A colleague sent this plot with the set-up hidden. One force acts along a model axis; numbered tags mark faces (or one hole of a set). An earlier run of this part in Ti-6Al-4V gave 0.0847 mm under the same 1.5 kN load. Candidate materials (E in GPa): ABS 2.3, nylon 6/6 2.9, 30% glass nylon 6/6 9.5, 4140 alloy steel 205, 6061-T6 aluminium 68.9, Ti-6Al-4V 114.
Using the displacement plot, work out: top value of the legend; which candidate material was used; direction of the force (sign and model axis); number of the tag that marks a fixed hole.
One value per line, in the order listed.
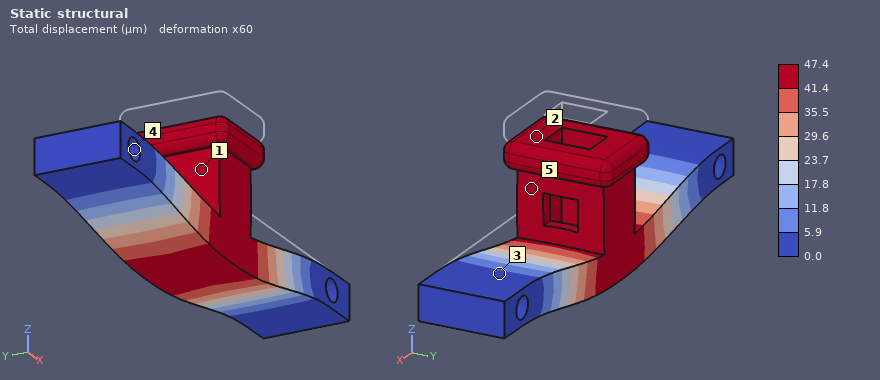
47.4 µm
4140 alloy steel
-Z
4
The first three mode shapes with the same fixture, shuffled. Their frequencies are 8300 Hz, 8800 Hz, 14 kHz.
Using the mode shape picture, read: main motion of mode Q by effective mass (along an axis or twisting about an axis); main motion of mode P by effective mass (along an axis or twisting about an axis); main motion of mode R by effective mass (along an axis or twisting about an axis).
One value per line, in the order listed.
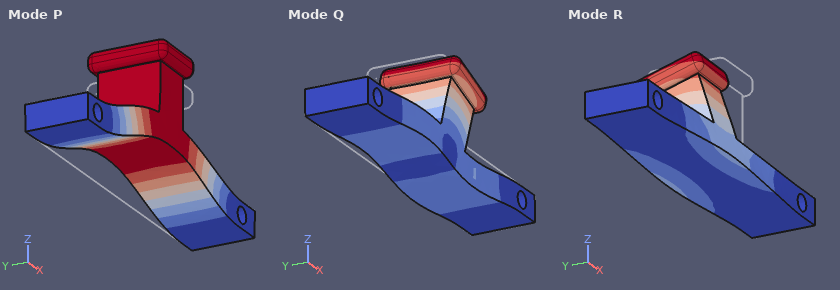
along X
along Z
along Y
